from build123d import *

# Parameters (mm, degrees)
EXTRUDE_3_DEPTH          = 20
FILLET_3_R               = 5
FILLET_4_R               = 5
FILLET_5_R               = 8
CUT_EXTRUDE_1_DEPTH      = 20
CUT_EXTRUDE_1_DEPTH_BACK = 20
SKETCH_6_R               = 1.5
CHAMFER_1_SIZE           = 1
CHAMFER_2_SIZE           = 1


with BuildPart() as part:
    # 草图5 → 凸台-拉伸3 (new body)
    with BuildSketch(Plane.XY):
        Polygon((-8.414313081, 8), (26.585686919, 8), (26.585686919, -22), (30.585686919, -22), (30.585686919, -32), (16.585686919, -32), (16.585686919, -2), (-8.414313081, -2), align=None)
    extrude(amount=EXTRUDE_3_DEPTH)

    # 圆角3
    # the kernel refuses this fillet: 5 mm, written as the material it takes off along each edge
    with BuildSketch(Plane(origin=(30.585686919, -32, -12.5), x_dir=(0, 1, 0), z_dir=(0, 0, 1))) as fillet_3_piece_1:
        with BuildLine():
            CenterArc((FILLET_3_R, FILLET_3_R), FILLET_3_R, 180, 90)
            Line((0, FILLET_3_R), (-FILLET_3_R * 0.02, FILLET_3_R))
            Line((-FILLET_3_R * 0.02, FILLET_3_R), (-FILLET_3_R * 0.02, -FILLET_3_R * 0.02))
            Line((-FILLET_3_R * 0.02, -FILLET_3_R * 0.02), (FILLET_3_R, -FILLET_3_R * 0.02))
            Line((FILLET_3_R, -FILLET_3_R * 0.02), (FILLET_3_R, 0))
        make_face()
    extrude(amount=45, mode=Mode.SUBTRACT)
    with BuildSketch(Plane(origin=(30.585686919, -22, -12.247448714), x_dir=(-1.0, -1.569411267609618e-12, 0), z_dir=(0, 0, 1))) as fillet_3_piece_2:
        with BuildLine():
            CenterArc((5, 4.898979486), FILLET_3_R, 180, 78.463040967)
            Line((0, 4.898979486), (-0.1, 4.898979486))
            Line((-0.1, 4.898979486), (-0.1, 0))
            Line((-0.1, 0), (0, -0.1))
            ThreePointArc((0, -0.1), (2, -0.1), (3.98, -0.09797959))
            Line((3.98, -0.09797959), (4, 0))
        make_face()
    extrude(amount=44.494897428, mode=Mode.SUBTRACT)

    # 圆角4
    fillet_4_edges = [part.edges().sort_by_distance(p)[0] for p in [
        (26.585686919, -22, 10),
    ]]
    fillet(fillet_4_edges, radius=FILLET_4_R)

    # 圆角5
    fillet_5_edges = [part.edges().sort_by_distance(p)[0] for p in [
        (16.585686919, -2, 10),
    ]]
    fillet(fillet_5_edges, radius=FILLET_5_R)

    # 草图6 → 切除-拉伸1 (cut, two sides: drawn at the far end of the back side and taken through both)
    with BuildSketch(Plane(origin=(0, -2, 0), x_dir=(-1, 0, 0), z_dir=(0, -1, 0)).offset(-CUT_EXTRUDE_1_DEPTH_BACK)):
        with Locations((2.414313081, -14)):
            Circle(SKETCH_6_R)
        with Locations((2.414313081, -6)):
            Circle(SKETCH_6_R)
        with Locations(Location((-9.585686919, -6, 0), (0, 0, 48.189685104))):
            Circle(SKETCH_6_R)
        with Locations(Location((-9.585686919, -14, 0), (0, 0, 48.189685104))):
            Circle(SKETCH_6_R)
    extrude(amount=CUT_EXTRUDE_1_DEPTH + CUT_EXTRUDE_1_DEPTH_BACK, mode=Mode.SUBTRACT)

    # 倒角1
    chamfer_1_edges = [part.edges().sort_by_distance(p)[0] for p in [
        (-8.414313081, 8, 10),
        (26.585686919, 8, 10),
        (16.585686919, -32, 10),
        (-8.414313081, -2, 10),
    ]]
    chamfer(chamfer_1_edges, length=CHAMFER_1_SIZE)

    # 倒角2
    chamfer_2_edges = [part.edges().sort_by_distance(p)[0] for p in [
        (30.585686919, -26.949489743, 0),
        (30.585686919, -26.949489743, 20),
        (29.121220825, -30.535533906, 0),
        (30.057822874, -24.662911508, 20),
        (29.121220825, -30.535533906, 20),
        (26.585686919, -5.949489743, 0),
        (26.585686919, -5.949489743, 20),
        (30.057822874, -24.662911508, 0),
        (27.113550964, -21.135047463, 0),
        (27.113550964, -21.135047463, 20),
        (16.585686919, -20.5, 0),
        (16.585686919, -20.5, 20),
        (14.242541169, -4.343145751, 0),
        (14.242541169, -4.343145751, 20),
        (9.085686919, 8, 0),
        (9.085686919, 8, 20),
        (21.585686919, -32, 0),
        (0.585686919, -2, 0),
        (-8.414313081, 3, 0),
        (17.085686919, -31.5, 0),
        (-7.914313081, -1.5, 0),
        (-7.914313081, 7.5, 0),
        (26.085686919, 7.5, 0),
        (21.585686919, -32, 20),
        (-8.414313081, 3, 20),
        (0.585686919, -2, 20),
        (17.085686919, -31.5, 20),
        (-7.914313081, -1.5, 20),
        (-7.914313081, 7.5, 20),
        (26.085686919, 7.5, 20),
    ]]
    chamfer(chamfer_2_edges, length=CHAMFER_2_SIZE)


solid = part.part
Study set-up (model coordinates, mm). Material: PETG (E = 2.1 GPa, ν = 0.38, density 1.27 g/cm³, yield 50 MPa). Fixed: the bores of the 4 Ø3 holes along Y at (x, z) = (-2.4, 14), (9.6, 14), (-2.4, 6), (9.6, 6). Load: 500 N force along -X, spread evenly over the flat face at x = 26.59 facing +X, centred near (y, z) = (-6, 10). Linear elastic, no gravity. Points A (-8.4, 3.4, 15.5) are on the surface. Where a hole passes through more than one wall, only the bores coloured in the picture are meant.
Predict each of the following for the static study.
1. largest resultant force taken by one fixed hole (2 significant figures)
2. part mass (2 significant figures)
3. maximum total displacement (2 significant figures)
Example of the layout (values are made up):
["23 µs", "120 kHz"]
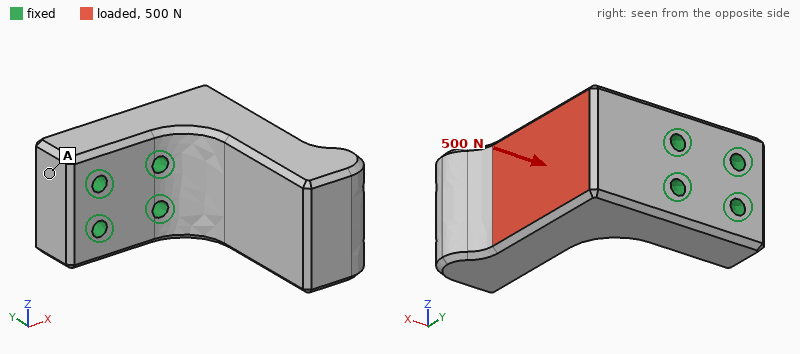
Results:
["240 N", "17 g", "0.41 mm"]
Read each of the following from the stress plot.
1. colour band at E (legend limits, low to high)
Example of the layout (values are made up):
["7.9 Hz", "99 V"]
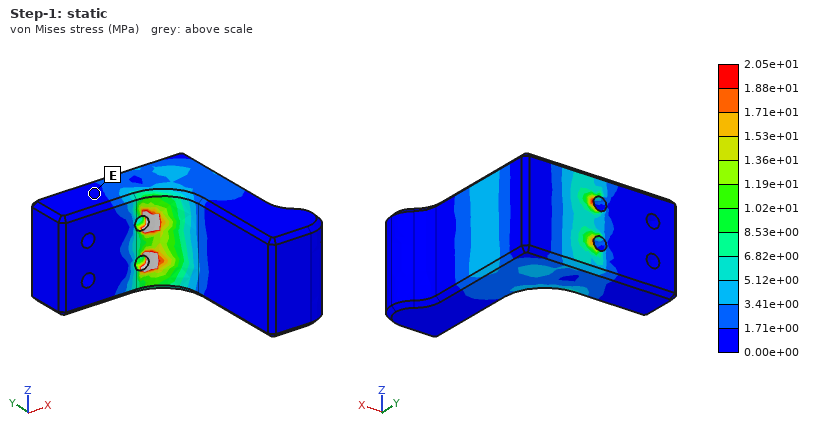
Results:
["0.00e+00 to 1.71e+00 MPa"]
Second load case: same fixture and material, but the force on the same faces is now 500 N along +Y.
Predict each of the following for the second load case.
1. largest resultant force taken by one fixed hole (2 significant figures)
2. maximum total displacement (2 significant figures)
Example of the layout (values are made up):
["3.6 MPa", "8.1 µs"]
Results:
["290 N", "0.63 mm"]
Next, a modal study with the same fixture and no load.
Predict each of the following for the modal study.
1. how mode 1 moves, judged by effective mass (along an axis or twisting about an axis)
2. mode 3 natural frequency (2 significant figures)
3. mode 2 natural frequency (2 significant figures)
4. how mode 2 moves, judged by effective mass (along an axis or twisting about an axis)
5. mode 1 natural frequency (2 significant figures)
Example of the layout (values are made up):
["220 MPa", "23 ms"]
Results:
["along X", "4000 Hz", "1700 Hz", "along Z", "1300 Hz"]
